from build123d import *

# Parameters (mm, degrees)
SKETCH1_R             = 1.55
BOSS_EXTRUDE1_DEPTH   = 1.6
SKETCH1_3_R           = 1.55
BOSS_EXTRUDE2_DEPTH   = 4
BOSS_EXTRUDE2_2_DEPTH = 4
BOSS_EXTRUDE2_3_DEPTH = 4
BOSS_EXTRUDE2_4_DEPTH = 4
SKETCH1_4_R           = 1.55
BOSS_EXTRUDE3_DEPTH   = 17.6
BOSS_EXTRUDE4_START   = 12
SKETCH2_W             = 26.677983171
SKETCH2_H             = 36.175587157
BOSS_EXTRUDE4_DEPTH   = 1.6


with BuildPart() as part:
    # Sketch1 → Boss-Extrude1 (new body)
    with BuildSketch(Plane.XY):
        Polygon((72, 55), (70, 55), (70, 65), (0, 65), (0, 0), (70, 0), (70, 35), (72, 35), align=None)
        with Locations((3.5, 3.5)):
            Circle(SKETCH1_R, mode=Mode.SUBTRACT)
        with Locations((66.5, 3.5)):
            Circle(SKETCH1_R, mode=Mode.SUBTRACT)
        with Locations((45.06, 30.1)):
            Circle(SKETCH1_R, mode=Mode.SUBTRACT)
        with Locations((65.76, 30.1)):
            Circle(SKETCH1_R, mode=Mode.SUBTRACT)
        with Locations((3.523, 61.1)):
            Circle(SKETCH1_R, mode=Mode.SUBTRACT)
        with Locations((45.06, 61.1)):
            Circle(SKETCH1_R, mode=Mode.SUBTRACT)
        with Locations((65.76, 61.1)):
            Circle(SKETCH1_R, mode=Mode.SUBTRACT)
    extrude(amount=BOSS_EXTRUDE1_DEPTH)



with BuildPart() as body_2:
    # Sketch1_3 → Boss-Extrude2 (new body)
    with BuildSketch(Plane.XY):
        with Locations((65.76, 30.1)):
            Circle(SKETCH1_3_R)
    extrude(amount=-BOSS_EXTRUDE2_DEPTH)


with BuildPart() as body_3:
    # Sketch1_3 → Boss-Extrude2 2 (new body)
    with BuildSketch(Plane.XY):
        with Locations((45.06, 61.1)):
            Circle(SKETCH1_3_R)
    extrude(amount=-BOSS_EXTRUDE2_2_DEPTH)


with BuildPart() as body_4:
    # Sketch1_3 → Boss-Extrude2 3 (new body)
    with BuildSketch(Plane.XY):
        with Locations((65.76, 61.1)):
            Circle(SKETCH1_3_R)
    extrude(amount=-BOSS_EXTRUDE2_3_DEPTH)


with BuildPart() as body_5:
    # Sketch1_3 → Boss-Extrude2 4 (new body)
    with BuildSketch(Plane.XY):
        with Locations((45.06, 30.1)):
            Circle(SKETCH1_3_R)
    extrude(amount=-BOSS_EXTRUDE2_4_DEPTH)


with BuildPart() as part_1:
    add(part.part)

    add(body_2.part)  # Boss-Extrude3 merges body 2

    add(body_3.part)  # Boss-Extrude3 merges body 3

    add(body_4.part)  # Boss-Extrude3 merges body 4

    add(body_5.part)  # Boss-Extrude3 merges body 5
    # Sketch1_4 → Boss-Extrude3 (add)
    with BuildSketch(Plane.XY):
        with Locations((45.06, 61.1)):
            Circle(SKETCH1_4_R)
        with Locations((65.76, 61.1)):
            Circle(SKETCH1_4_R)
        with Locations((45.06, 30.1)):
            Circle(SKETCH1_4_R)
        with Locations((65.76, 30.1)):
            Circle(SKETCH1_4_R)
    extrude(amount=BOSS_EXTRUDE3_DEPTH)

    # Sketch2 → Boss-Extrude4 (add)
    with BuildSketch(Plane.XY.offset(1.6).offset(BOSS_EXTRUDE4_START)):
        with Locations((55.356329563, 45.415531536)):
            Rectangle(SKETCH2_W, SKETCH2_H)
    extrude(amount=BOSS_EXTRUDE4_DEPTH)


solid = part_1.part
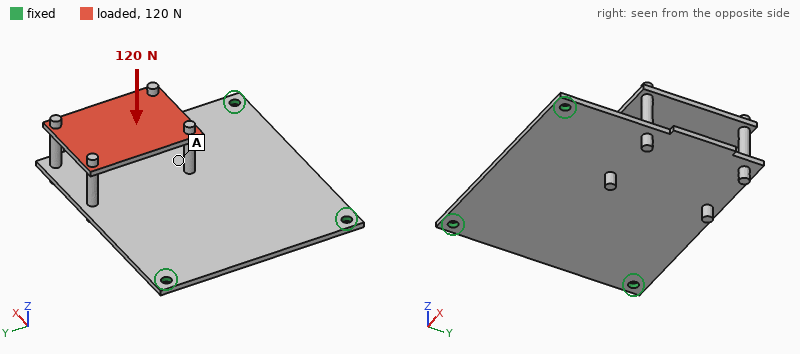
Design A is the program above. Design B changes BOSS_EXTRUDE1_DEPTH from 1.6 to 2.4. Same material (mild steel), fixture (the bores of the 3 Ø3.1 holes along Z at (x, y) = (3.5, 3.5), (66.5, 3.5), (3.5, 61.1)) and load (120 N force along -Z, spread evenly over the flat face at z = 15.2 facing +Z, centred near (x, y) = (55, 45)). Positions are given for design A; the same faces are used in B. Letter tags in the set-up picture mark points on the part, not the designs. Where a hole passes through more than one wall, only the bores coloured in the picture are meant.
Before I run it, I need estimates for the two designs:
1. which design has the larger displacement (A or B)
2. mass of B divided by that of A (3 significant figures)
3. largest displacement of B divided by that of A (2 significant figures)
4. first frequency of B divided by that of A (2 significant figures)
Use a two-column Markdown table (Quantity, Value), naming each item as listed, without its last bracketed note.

| Quantity | Value |
|---|---|
| which design has the larger displacement | A |
| mass of B divided by that of A | 1.39 |
| largest displacement of B divided by that of A | 0.35 |
| first frequency of B divided by that of A | 1.5 |
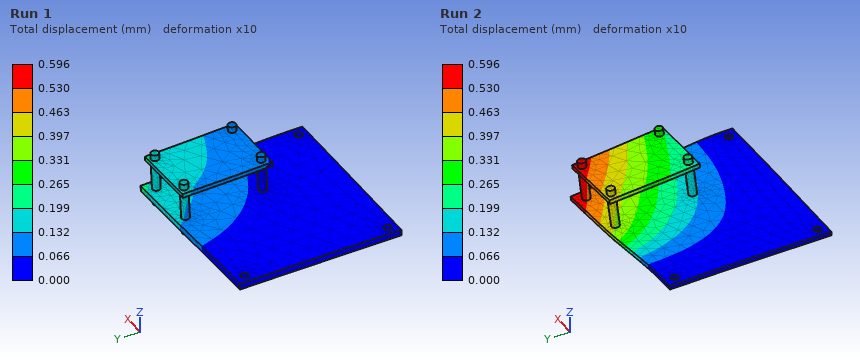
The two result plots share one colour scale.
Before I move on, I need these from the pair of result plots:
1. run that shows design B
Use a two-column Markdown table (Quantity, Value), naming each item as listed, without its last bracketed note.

| Quantity | Value |
|---|---|
| run that shows design B | Run 1 |
